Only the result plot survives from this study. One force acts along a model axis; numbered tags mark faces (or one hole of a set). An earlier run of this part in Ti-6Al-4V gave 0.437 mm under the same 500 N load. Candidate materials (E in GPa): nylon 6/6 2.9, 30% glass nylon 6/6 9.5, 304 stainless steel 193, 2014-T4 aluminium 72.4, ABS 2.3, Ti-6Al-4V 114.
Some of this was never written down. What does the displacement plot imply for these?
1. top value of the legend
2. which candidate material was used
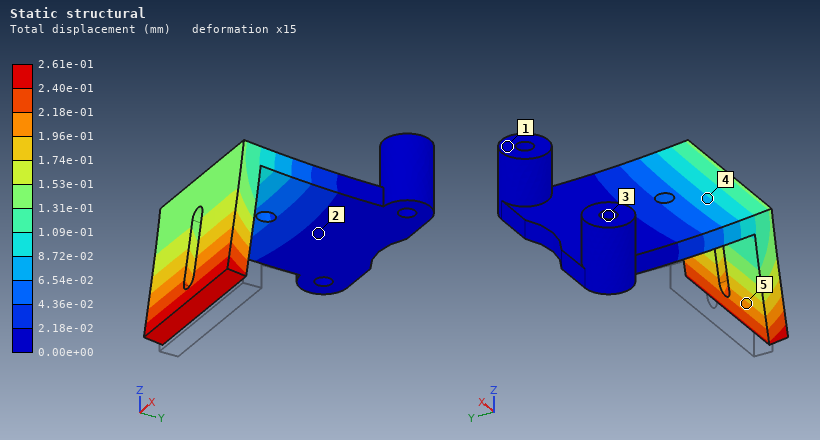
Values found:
2.61e-01 mm
304 stainless steel
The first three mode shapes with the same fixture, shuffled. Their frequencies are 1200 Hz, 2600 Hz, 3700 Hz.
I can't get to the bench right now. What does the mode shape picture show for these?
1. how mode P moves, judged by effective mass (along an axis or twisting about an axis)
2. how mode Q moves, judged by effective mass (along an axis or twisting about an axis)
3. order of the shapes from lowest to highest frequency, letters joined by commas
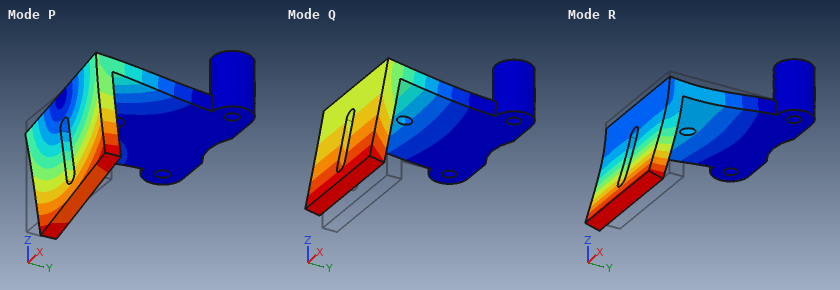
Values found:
along X
along Z
Q, P, R
